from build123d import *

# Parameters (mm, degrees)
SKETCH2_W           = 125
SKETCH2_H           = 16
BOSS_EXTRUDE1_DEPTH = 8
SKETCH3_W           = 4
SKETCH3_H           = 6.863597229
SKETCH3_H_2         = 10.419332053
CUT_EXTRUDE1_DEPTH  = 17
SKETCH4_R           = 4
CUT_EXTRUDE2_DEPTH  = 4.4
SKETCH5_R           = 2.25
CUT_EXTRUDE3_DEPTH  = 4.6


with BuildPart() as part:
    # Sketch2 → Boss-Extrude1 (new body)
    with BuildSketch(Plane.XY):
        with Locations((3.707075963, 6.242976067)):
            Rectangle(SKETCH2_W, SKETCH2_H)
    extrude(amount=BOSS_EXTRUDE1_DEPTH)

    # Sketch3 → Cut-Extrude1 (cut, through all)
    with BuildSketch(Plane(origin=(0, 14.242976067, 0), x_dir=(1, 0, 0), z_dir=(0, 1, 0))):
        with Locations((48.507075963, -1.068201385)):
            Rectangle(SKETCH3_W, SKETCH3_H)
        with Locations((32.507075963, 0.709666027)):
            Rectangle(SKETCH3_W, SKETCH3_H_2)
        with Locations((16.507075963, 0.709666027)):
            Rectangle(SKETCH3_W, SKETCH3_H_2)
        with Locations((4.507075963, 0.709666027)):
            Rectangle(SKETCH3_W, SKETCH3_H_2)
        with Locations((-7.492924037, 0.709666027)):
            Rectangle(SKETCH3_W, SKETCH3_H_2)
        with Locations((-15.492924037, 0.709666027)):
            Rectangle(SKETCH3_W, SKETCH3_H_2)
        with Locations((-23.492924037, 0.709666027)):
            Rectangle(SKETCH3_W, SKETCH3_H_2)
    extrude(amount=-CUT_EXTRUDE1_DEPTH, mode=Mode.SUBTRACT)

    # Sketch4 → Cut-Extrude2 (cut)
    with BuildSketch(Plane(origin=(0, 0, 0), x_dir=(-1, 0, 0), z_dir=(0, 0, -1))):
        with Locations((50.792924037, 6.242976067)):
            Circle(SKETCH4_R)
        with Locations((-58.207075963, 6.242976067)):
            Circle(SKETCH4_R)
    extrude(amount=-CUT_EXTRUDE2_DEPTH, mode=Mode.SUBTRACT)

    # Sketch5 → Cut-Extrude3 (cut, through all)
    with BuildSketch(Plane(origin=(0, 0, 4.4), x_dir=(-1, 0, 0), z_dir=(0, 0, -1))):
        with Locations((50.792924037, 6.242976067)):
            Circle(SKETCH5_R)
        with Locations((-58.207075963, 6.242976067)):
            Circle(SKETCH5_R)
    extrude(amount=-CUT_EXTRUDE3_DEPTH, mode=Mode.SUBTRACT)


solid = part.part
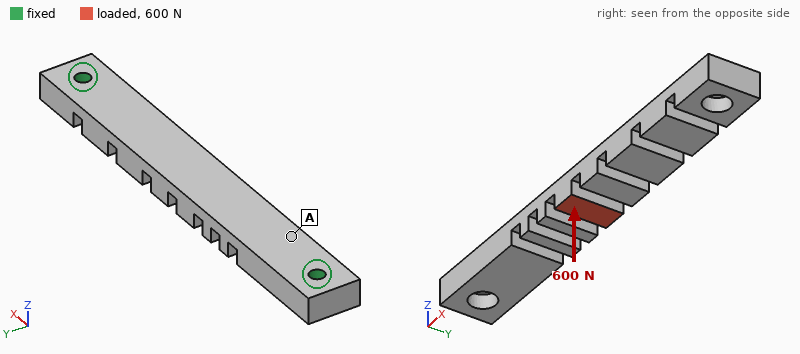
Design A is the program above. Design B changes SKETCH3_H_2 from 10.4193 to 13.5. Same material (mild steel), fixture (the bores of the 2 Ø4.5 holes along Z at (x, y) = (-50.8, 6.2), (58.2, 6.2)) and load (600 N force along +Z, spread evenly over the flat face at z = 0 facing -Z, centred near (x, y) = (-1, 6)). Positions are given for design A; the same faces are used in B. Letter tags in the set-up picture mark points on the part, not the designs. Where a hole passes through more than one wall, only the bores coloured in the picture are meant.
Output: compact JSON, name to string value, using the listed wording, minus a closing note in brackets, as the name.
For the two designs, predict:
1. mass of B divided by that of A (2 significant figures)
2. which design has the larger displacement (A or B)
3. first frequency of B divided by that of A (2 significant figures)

{"mass of B divided by that of A": "0.96", "which design has the larger displacement": "B", "first frequency of B divided by that of A": "0.76"}
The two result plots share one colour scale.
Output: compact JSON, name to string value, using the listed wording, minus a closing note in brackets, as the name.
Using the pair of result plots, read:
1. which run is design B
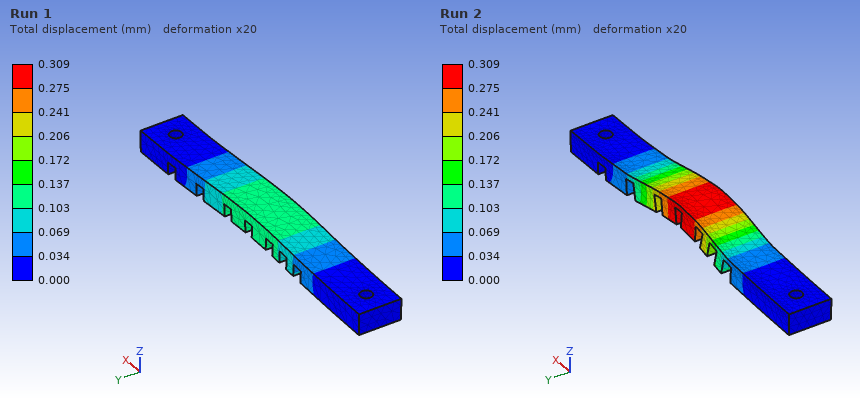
{"which run is design B": "Run 2"}
